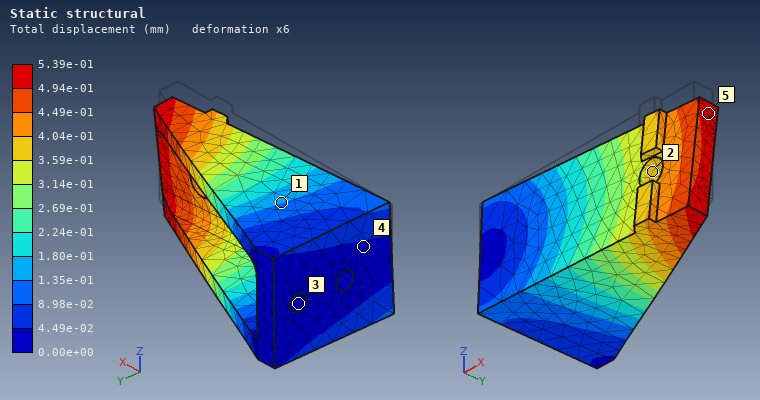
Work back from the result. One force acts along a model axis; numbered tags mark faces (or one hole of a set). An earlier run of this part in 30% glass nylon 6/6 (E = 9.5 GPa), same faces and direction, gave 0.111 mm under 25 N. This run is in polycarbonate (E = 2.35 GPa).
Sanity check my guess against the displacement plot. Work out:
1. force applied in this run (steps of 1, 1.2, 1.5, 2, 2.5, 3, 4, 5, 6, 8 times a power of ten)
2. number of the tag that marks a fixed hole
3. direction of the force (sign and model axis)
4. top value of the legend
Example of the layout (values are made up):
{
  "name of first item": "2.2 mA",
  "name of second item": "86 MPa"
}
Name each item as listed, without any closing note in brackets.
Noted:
{
  "force applied in this run": "30 N",
  "number of the tag that marks a fixed hole": "3",
  "direction of the force": "-Z",
  "top value of the legend": "5.39e-01 mm"
}
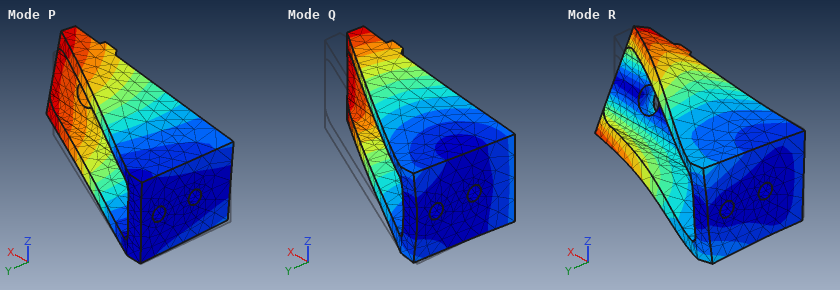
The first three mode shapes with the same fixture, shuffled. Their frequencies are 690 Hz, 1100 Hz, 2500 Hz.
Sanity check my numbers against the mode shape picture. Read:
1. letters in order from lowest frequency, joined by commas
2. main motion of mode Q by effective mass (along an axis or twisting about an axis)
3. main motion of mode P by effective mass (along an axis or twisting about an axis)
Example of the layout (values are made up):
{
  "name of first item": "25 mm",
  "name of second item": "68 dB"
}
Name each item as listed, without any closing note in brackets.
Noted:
{
  "letters in order from lowest frequency, joined by commas": "P, Q, R",
  "main motion of mode Q by effective mass": "along Y",
  "main motion of mode P by effective mass": "along Z"
}
